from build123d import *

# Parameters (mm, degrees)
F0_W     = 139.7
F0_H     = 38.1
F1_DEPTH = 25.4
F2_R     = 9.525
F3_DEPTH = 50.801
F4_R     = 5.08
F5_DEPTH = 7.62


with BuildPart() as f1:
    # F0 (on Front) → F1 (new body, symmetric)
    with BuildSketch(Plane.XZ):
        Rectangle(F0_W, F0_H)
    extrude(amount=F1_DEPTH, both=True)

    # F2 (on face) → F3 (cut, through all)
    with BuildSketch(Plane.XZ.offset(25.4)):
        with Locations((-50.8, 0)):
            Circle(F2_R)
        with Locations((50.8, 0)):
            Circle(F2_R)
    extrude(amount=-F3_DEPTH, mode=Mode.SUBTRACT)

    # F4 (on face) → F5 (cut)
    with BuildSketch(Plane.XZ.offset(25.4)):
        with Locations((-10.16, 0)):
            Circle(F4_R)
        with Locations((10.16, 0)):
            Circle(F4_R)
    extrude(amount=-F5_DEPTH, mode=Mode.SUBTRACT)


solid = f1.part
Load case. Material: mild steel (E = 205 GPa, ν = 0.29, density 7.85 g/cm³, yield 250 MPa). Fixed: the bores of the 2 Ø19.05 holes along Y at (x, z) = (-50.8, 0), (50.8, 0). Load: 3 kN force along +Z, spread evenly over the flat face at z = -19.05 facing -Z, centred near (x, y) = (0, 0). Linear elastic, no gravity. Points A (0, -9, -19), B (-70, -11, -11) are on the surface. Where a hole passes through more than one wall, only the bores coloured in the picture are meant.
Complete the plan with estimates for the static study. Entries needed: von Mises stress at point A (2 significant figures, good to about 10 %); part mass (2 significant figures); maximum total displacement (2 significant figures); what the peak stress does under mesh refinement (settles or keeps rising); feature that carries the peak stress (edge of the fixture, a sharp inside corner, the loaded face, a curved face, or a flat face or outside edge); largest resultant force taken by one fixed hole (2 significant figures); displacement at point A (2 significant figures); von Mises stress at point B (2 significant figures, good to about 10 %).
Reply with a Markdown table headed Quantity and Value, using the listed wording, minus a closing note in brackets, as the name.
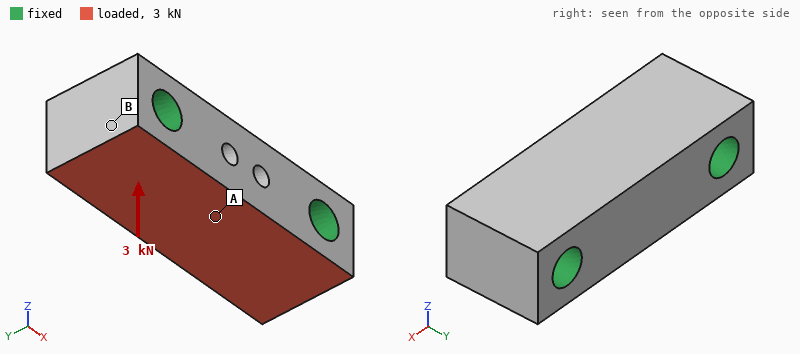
| Quantity | Value |
|---|---|
| von Mises stress at point A | 0.89 MPa |
| part mass | 1.9 kg |
| maximum total displacement | 0.33 µm |
| what the peak stress does under mesh refinement | keeps rising |
| feature that carries the peak stress | edge of the fixture |
| largest resultant force taken by one fixed hole | 1.5 kN |
| displacement at point A | 0.30 µm |
| von Mises stress at point B | 0.32 MPa |
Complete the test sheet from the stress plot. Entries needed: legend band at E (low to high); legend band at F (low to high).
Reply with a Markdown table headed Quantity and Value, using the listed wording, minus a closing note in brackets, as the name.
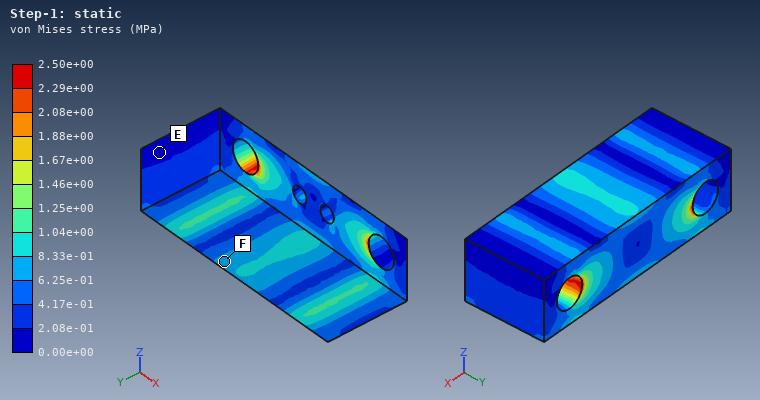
| Quantity | Value |
|---|---|
| legend band at E | 0.00e+00 to 2.08e-01 MPa |
| legend band at F | 6.25e-01 to 8.33e-01 MPa |
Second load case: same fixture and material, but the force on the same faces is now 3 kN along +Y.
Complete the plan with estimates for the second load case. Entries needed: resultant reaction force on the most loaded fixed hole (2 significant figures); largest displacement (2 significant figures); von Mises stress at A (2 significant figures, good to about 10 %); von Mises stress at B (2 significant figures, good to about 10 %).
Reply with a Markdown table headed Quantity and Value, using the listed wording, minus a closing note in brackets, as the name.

| Quantity | Value |
|---|---|
| resultant reaction force on the most loaded fixed hole | 1.5 kN |
| largest displacement | 0.59 µm |
| von Mises stress at A | 0.82 MPa |
| von Mises stress at B | 0.62 MPa |
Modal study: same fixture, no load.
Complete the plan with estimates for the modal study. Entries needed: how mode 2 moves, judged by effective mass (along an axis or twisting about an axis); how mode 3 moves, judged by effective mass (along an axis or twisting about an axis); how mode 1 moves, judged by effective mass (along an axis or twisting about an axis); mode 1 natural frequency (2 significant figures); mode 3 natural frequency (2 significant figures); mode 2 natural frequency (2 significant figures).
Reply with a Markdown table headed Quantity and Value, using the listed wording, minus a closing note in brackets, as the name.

| Quantity | Value |
|---|---|
| how mode 2 moves, judged by effective mass | along Y |
| how mode 3 moves, judged by effective mass | twisting about X |
| how mode 1 moves, judged by effective mass | along Z |
| mode 1 natural frequency | 13 kHz |
| mode 3 natural frequency | 16 kHz |
| mode 2 natural frequency | 15 kHz |
